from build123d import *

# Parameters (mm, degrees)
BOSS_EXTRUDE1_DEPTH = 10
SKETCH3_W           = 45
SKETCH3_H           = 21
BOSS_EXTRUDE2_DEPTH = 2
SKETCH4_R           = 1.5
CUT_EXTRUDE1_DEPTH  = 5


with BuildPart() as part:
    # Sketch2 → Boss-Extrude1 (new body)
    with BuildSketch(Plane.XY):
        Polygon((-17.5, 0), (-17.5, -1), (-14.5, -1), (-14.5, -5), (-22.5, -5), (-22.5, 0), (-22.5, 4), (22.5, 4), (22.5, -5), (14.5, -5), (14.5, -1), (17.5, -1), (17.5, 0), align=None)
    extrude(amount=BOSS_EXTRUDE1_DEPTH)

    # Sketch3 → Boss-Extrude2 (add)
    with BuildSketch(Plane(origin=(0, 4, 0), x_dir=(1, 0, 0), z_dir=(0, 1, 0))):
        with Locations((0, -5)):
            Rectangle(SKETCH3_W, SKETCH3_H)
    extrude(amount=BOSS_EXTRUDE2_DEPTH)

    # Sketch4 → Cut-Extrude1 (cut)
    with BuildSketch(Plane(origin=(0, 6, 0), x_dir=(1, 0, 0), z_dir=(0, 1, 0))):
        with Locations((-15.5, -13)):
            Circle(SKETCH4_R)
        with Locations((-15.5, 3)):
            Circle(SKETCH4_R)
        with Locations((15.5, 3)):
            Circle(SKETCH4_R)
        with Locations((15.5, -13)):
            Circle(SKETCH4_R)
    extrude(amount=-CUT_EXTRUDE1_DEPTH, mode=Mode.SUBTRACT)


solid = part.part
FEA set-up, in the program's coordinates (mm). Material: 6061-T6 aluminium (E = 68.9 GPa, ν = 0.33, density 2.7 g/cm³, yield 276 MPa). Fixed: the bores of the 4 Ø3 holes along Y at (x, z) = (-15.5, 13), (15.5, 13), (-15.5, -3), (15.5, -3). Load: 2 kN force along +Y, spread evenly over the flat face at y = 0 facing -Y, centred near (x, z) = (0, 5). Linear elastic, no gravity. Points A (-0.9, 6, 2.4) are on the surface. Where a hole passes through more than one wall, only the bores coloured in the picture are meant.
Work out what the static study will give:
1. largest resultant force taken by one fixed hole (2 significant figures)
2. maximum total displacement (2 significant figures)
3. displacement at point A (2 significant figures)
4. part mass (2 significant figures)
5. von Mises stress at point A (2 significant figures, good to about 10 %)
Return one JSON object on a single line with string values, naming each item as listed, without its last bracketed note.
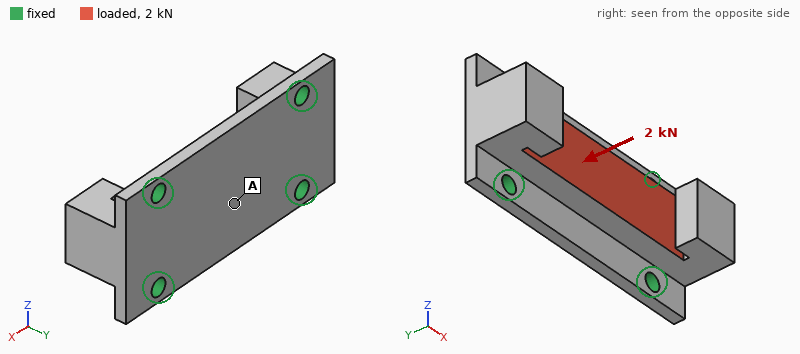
{"largest resultant force taken by one fixed hole": "630 N", "maximum total displacement": "32 µm", "displacement at point A": "31 µm", "part mass": "12 g", "von Mises stress at point A": "41 MPa"}
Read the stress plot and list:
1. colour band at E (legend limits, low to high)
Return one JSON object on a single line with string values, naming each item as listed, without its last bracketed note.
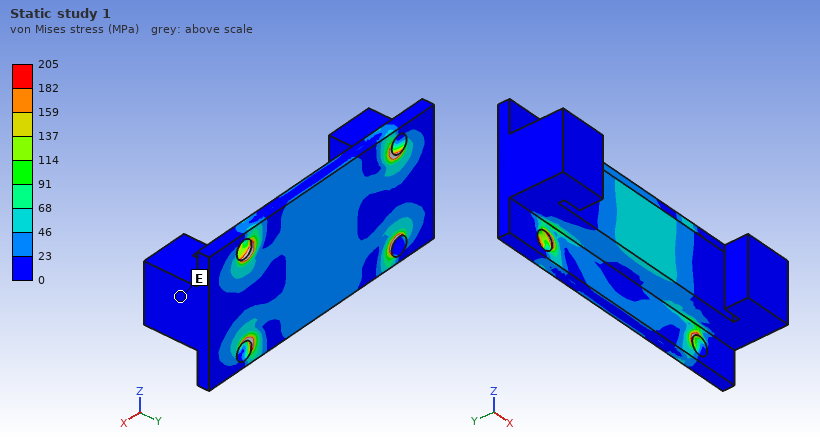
{"colour band at E": "0 to 23 MPa"}
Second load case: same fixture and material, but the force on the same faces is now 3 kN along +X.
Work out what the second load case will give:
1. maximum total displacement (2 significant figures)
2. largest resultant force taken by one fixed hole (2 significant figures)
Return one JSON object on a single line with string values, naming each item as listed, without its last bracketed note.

{"maximum total displacement": "17 µm", "largest resultant force taken by one fixed hole": "800 N"}
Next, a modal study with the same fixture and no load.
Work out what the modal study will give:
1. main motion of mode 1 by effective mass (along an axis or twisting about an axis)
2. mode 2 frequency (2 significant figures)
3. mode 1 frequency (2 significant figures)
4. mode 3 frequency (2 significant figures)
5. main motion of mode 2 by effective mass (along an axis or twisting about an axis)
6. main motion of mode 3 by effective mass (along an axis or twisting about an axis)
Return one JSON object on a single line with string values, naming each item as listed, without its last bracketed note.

{"main motion of mode 1 by effective mass": "along Y", "mode 2 frequency": "20 kHz", "mode 1 frequency": "15 kHz", "mode 3 frequency": "23 kHz", "main motion of mode 2 by effective mass": "along X", "main motion of mode 3 by effective mass": "along Y"}
